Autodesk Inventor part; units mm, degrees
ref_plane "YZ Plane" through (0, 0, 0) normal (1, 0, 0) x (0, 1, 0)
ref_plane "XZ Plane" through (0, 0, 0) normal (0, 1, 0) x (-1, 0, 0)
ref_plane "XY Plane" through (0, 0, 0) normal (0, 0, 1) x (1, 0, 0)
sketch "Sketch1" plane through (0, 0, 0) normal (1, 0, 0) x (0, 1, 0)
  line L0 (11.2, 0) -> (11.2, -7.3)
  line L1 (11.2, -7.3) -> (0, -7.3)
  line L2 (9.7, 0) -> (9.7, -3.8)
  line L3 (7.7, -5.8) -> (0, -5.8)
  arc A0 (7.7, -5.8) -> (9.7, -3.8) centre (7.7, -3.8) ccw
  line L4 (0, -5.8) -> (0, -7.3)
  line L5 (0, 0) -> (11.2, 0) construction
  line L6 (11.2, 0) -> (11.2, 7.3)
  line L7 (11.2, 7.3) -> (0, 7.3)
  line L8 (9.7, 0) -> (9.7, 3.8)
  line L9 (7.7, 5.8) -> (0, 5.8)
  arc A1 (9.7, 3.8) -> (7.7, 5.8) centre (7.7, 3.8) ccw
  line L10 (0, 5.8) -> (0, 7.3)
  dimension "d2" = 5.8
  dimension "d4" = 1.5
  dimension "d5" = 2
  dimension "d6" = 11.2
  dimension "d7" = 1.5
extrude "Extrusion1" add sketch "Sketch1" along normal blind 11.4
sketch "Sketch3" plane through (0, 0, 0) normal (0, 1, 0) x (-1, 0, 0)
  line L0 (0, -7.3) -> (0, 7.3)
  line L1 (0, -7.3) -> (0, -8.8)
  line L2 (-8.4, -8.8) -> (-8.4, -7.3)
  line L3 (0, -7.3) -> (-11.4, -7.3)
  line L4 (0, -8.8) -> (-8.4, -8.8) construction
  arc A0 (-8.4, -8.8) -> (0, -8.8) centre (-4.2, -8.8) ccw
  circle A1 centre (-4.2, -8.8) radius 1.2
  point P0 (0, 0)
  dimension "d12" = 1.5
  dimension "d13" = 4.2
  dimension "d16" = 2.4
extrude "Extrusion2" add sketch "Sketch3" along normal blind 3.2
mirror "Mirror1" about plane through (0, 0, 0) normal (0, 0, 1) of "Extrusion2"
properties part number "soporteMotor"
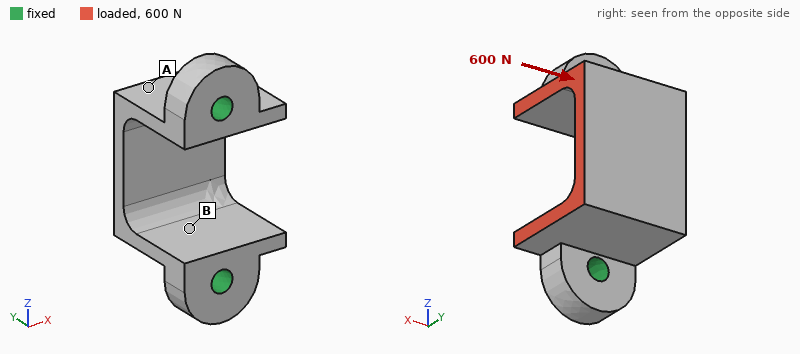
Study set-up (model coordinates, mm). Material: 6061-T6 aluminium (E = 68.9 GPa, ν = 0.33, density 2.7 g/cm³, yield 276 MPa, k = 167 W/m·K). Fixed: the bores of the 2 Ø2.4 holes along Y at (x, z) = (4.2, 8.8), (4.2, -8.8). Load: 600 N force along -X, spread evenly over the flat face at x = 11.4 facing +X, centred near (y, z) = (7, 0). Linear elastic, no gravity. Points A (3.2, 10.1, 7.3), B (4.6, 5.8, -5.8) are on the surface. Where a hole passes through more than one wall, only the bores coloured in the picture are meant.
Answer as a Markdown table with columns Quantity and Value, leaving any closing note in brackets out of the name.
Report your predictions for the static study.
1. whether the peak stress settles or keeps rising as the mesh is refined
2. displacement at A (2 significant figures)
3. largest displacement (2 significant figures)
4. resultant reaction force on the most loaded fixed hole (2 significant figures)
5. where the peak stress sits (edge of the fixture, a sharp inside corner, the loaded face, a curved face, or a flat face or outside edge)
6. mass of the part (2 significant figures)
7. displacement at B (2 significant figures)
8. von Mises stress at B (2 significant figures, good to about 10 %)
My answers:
| Quantity | Value |
|---|---|
| whether the peak stress settles or keeps rising as the mesh is refined | keeps rising |
| displacement at A | 23 µm |
| largest displacement | 33 µm |
| resultant reaction force on the most loaded fixed hole | 300 N |
| where the peak stress sits | edge of the fixture |
| mass of the part | 2.2 g |
| displacement at B | 11 µm |
| von Mises stress at B | 39 MPa |
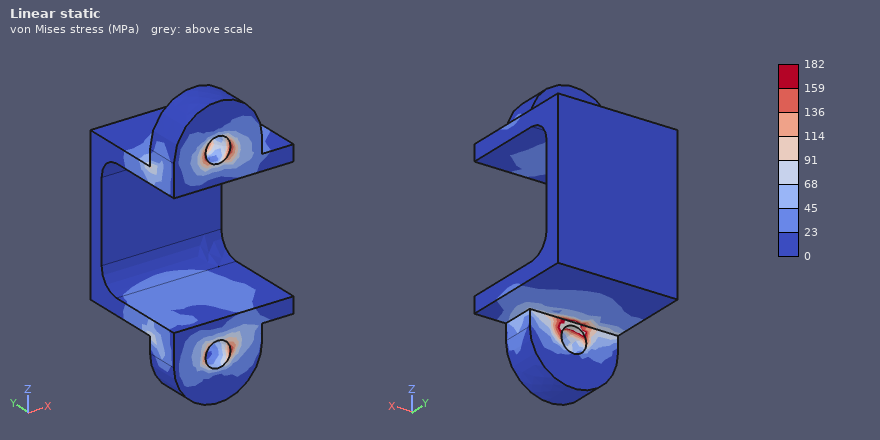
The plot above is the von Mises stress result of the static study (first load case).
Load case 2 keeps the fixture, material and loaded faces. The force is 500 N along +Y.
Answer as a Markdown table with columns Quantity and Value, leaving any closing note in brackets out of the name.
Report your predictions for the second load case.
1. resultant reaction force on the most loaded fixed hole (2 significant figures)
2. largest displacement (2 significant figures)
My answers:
| Quantity | Value |
|---|---|
| resultant reaction force on the most loaded fixed hole | 250 N |
| largest displacement | 50 µm |
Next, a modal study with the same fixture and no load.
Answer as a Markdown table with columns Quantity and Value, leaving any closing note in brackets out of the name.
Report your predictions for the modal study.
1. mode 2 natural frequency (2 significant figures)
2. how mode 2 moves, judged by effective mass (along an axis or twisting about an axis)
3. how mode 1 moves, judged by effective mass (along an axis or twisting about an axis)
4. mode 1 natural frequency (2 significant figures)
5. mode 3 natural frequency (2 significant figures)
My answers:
| Quantity | Value |
|---|---|
| mode 2 natural frequency | 19 kHz |
| how mode 2 moves, judged by effective mass | along X |
| how mode 1 moves, judged by effective mass | along Z |
| mode 1 natural frequency | 15 kHz |
| mode 3 natural frequency | 24 kHz |
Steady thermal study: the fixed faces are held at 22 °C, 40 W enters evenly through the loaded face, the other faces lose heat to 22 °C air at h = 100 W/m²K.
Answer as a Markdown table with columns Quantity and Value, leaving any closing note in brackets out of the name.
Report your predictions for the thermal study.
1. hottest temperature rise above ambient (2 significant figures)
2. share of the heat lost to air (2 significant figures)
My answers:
| Quantity | Value |
|---|---|
| hottest temperature rise above ambient | 67 K |
| share of the heat lost to air | 7.2 % |
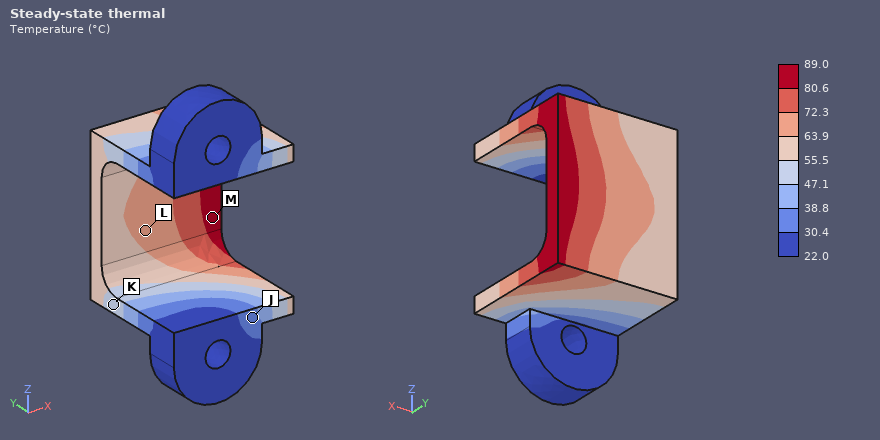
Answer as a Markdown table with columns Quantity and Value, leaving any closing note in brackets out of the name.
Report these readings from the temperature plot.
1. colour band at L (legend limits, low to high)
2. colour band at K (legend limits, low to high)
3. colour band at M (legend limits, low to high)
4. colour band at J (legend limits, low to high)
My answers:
| Quantity | Value |
|---|---|
| colour band at L | 63.9 to 72.3 °C |
| colour band at K | 47.1 to 55.5 °C |
| colour band at M | 80.6 to 89.0 °C |
| colour band at J | 30.4 to 38.8 °C |
